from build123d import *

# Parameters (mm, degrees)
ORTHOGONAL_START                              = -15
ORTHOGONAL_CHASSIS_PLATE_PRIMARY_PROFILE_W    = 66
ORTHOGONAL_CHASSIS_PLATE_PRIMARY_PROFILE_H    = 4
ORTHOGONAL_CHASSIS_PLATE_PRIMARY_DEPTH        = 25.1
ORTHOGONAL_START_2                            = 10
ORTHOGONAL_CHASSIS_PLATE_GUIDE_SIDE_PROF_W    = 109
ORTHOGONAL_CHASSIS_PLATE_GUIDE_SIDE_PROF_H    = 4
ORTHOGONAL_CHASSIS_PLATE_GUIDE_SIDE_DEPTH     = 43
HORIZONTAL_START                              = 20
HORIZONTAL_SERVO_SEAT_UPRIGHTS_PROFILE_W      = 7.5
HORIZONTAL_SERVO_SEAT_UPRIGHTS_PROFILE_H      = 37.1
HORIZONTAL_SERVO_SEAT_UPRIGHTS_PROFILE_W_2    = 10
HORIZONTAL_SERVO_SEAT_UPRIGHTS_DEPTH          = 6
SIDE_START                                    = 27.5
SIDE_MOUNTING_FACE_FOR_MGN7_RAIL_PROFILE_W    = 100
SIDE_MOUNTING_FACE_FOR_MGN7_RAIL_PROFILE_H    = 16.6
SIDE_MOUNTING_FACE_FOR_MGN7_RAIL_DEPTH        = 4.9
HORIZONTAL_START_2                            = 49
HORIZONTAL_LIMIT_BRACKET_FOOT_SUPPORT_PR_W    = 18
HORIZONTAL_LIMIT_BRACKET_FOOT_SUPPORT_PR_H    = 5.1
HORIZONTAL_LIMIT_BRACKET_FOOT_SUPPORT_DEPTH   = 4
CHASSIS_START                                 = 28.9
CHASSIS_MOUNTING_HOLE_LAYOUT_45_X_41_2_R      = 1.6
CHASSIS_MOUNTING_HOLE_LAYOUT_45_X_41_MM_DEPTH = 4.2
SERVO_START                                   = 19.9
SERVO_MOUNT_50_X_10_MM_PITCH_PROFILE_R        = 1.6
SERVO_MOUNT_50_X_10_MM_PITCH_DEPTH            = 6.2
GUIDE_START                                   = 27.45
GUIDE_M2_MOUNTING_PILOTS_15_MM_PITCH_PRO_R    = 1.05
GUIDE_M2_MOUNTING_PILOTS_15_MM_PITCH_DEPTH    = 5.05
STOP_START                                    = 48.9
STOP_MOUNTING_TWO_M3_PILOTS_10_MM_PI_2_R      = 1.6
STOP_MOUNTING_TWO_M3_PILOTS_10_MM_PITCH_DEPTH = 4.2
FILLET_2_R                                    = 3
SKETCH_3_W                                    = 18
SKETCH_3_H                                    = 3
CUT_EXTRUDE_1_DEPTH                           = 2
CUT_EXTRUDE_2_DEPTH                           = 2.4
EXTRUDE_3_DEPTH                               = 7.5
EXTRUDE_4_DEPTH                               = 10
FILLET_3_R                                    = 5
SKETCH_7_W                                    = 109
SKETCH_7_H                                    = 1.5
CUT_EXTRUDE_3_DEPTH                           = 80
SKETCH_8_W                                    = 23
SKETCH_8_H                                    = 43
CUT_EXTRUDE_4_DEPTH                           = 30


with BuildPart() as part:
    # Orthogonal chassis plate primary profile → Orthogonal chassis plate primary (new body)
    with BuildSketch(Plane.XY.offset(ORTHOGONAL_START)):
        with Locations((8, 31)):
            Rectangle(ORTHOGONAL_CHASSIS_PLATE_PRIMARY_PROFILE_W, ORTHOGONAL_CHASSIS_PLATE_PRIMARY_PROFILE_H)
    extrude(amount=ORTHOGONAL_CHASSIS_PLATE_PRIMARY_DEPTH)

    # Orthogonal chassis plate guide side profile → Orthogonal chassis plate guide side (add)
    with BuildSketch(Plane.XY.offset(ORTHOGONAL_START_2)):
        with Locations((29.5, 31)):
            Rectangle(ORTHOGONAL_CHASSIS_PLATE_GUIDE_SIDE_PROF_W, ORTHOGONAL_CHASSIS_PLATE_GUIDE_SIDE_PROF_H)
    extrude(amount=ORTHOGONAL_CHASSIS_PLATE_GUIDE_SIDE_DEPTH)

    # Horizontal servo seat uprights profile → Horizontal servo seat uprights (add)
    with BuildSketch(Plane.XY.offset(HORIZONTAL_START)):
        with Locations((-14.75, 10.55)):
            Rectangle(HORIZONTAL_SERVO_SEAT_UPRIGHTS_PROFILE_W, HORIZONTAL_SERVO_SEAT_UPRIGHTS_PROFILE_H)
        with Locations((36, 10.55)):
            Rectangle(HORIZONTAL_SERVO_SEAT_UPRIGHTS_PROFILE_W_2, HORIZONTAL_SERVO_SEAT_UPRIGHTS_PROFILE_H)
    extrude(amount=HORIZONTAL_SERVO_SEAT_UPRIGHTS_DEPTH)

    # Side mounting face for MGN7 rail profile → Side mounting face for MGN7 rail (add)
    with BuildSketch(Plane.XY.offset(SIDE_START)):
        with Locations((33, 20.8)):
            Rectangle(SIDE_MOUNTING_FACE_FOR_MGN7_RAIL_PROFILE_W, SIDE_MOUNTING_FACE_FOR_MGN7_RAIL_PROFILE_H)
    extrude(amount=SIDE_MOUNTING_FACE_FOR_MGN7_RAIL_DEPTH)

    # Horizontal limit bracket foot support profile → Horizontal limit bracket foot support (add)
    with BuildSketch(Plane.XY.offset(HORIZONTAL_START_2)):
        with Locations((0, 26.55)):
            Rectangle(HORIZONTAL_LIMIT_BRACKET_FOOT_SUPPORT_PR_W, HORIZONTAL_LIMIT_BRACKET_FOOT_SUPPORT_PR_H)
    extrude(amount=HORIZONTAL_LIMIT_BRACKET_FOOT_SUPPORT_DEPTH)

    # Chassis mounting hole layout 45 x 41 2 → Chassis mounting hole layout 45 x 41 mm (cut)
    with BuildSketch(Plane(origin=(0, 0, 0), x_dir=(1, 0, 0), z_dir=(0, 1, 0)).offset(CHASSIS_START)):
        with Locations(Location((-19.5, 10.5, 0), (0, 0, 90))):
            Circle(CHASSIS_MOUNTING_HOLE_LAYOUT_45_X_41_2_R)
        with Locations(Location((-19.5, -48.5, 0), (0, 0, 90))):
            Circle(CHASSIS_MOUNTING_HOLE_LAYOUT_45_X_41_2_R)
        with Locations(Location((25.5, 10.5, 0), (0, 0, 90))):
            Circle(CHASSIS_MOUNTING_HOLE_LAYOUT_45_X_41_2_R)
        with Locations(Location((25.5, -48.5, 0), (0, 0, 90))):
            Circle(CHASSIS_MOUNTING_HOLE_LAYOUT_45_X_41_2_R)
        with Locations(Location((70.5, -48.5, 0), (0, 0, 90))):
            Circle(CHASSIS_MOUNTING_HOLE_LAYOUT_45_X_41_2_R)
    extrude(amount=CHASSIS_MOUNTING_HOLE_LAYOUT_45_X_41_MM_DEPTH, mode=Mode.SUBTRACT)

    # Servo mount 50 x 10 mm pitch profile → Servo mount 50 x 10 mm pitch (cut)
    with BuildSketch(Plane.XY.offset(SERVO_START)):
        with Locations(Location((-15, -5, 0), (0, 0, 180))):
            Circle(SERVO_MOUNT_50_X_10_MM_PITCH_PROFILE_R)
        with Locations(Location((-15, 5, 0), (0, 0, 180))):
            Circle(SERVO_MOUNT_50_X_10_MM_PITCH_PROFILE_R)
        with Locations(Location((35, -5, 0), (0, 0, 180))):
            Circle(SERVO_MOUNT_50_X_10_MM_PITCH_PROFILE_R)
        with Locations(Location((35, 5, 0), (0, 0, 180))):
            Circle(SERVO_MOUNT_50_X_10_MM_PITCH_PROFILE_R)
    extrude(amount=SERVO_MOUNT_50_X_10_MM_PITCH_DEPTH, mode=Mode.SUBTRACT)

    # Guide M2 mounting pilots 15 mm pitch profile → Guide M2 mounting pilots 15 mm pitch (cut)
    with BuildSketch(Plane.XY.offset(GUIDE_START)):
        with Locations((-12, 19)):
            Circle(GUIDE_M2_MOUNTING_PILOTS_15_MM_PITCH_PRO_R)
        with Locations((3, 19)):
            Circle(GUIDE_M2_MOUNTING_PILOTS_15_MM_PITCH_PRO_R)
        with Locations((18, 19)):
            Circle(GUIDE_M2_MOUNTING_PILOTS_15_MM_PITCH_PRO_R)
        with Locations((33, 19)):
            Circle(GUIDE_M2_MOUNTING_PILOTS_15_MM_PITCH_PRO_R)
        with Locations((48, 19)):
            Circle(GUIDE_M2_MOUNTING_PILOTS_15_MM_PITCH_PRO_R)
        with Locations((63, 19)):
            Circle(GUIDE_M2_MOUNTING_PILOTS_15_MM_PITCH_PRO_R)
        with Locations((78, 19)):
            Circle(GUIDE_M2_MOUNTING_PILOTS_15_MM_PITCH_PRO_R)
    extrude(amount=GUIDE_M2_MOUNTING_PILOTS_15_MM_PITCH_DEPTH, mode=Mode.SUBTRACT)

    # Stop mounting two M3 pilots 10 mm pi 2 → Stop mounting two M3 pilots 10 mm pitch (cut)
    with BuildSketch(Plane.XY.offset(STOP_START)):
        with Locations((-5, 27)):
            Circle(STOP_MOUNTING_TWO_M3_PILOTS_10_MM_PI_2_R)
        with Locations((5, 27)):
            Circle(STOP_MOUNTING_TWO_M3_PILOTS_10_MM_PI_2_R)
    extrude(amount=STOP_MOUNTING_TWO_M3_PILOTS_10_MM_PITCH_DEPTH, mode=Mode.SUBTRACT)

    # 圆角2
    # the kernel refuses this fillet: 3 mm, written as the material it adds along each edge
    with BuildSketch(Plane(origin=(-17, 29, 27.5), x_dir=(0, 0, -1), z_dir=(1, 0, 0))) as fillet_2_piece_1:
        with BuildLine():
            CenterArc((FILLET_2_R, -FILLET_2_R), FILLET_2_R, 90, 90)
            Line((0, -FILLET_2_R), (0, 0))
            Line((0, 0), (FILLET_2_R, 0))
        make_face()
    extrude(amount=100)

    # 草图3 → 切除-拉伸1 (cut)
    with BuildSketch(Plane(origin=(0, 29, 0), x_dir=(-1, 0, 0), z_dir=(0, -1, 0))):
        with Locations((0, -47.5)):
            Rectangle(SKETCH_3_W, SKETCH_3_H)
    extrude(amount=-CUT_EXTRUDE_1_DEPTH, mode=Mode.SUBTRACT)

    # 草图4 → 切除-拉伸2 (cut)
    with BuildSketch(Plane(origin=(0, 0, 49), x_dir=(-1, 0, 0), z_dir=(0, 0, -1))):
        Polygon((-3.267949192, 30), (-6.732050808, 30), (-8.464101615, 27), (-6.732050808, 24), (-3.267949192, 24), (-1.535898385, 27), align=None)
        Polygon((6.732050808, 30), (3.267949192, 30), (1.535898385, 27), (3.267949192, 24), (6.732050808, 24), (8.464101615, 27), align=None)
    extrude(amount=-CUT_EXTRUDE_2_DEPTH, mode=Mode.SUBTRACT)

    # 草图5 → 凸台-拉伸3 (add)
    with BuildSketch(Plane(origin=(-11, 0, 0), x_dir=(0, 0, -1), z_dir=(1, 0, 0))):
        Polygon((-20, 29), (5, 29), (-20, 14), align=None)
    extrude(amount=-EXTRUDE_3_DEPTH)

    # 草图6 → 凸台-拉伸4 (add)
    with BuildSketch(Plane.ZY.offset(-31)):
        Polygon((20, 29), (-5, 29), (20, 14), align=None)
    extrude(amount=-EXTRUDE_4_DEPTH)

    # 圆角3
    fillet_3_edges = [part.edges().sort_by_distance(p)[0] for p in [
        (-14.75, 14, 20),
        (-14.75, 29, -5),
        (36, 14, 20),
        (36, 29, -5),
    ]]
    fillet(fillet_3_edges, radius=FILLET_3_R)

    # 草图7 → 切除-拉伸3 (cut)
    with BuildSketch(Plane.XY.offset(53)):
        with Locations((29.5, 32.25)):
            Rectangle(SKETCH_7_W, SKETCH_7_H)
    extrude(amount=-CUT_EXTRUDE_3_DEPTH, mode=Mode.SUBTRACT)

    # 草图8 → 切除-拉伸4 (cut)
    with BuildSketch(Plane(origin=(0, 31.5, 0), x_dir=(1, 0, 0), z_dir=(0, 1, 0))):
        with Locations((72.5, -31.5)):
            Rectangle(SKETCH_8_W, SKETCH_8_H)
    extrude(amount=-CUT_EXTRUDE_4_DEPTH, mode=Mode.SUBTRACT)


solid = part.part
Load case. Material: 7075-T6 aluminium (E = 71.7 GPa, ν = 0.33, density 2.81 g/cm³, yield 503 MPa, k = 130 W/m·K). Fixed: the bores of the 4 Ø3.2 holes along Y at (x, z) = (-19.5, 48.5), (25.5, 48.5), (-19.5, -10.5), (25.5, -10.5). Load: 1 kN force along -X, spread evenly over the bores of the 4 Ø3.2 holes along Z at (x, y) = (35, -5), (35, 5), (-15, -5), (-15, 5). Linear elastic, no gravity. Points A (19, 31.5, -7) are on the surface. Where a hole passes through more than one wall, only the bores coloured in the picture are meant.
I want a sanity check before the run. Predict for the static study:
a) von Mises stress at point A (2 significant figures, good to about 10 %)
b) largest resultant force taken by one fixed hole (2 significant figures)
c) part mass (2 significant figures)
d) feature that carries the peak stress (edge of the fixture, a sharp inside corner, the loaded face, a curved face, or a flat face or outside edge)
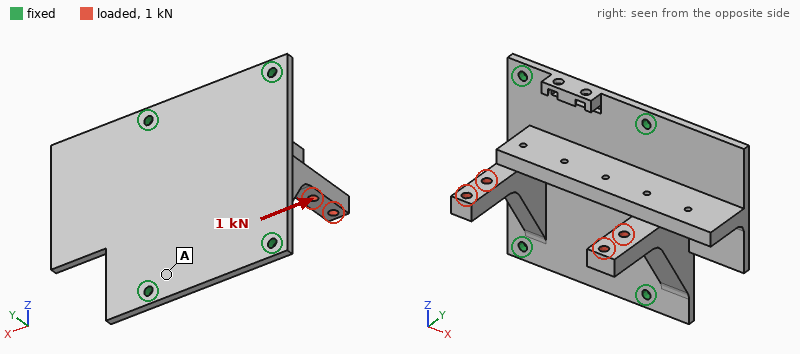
29 MPa
550 N
75 g
a flat face or outside edge
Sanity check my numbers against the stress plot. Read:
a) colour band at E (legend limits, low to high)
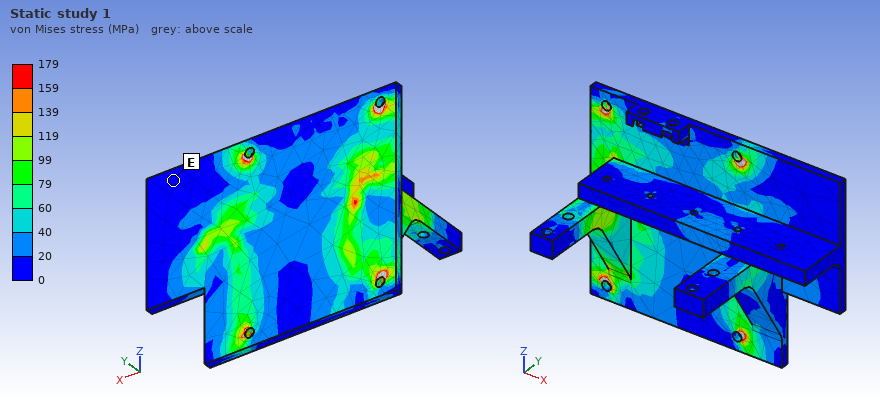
0 to 20 MPa
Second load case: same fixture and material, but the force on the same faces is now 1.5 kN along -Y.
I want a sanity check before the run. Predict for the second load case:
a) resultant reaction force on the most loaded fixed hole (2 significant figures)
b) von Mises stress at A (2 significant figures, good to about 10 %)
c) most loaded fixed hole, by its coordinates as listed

660 N
39 MPa
(25.5, 48.5)
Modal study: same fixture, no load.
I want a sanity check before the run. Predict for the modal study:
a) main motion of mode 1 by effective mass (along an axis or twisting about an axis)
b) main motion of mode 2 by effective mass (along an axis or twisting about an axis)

along Y
along Y
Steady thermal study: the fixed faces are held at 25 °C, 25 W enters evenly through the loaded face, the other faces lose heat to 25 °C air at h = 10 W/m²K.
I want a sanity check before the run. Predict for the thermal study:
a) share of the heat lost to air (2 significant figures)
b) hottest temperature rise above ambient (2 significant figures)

10 %
69 K
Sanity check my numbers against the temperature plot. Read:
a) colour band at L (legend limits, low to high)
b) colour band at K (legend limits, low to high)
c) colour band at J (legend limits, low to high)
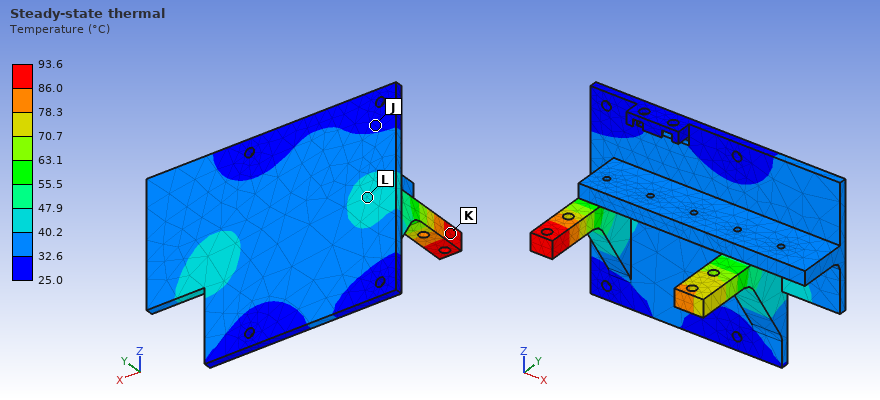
40.2 to 47.9 °C
86.0 to 93.6 °C
25.0 to 32.6 °C
